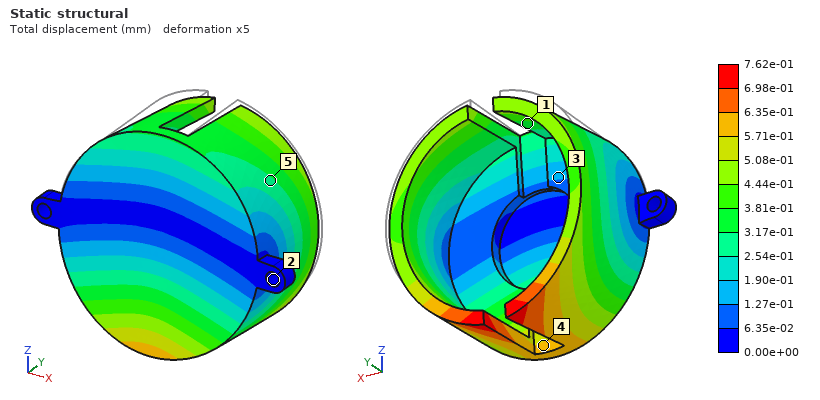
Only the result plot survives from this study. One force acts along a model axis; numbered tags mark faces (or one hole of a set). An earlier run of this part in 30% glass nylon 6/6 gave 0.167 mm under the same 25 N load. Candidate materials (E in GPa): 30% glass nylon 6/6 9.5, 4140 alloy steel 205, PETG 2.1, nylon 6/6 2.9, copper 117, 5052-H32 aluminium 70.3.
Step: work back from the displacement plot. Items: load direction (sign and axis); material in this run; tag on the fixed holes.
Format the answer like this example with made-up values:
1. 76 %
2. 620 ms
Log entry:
1. -Y
2. PETG
3. 2
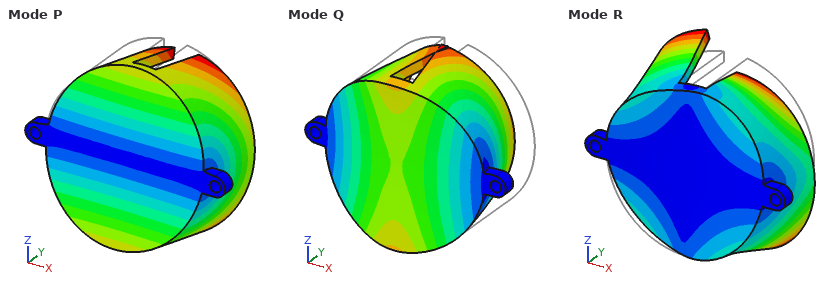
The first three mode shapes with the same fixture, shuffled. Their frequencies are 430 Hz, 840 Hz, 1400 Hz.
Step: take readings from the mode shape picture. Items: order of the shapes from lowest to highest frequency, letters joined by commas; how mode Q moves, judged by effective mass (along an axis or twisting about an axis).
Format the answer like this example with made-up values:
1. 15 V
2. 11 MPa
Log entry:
1. P, Q, R
2. along Y
